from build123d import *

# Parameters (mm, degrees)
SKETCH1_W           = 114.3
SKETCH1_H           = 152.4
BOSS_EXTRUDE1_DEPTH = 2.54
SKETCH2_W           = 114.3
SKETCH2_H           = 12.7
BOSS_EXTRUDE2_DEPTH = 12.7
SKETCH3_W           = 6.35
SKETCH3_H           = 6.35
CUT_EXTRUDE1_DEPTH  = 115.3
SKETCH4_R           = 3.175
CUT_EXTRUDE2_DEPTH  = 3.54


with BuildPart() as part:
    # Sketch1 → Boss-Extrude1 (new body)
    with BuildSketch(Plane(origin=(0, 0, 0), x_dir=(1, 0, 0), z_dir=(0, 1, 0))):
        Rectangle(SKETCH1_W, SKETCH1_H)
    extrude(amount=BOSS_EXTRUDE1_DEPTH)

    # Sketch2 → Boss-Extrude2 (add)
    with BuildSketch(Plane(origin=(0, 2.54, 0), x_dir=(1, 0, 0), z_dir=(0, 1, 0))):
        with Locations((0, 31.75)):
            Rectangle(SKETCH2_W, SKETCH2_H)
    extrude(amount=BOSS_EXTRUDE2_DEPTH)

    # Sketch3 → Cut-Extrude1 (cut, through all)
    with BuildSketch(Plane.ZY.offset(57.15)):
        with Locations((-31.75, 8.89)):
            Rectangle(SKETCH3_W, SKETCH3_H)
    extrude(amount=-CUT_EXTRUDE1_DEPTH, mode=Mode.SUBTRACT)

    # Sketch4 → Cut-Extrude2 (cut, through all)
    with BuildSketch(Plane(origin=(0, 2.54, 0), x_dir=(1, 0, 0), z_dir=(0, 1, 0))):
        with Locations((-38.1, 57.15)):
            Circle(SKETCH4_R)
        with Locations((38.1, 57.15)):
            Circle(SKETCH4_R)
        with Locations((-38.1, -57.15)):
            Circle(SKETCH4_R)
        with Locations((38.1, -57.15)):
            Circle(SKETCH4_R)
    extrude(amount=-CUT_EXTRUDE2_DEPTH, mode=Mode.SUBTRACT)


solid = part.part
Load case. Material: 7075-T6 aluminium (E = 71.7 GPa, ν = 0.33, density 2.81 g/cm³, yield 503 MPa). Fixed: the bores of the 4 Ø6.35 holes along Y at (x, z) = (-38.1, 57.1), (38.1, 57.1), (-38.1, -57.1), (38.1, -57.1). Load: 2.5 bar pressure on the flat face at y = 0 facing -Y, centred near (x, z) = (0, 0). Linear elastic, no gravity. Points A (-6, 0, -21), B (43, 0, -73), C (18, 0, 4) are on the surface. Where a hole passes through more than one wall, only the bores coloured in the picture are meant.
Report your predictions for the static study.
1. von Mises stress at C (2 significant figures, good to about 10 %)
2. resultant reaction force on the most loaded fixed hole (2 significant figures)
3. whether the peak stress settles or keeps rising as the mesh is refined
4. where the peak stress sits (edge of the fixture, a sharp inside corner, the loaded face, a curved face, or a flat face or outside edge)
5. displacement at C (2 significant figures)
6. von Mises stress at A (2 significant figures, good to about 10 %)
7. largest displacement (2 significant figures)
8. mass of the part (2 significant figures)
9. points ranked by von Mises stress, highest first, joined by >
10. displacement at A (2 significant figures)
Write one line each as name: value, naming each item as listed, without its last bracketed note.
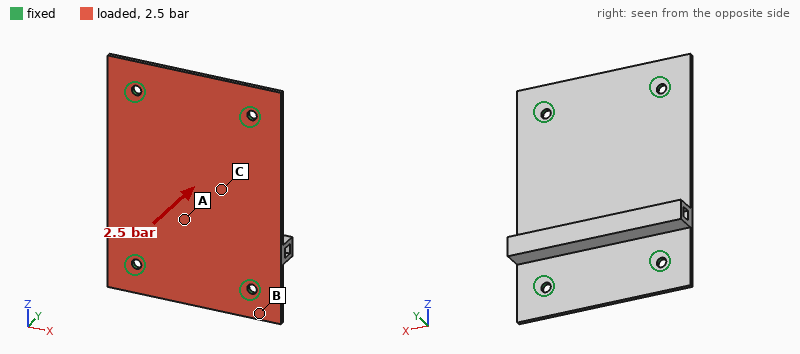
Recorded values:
von Mises stress at C: 120 MPa
resultant reaction force on the most loaded fixed hole: 1.1 kN
whether the peak stress settles or keeps rising as the mesh is refined: keeps rising
where the peak stress sits: edge of the fixture
displacement at C: 1.2 mm
von Mises stress at A: 65 MPa
largest displacement: 1.3 mm
mass of the part: 160 g
points ranked by von Mises stress, highest first, joined by >: C > A > B
displacement at A: 0.94 mm
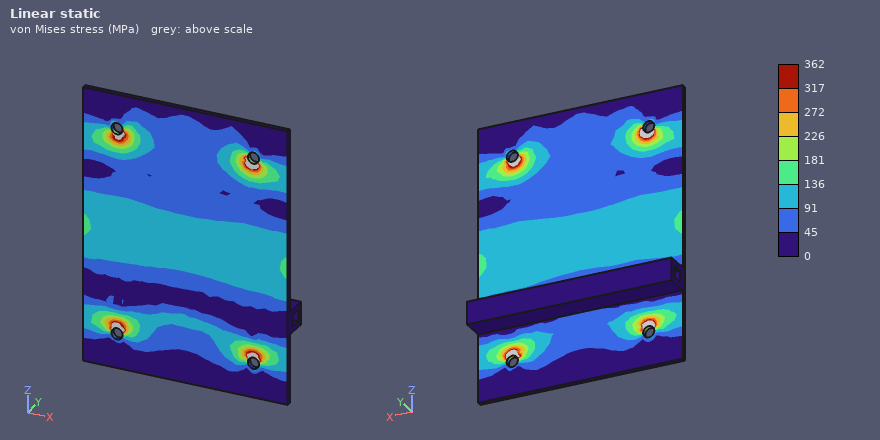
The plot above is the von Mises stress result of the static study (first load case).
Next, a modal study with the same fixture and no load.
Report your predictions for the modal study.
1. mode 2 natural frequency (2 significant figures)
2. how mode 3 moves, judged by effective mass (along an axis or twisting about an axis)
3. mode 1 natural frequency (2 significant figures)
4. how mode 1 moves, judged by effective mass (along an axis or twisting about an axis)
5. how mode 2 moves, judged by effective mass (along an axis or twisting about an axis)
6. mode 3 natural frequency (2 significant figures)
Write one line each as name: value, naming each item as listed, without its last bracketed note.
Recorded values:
mode 2 natural frequency: 1600 Hz
how mode 3 moves, judged by effective mass: twisting about X
mode 1 natural frequency: 830 Hz
how mode 1 moves, judged by effective mass: along Y
how mode 2 moves, judged by effective mass: twisting about Z
mode 3 natural frequency: 2100 Hz
